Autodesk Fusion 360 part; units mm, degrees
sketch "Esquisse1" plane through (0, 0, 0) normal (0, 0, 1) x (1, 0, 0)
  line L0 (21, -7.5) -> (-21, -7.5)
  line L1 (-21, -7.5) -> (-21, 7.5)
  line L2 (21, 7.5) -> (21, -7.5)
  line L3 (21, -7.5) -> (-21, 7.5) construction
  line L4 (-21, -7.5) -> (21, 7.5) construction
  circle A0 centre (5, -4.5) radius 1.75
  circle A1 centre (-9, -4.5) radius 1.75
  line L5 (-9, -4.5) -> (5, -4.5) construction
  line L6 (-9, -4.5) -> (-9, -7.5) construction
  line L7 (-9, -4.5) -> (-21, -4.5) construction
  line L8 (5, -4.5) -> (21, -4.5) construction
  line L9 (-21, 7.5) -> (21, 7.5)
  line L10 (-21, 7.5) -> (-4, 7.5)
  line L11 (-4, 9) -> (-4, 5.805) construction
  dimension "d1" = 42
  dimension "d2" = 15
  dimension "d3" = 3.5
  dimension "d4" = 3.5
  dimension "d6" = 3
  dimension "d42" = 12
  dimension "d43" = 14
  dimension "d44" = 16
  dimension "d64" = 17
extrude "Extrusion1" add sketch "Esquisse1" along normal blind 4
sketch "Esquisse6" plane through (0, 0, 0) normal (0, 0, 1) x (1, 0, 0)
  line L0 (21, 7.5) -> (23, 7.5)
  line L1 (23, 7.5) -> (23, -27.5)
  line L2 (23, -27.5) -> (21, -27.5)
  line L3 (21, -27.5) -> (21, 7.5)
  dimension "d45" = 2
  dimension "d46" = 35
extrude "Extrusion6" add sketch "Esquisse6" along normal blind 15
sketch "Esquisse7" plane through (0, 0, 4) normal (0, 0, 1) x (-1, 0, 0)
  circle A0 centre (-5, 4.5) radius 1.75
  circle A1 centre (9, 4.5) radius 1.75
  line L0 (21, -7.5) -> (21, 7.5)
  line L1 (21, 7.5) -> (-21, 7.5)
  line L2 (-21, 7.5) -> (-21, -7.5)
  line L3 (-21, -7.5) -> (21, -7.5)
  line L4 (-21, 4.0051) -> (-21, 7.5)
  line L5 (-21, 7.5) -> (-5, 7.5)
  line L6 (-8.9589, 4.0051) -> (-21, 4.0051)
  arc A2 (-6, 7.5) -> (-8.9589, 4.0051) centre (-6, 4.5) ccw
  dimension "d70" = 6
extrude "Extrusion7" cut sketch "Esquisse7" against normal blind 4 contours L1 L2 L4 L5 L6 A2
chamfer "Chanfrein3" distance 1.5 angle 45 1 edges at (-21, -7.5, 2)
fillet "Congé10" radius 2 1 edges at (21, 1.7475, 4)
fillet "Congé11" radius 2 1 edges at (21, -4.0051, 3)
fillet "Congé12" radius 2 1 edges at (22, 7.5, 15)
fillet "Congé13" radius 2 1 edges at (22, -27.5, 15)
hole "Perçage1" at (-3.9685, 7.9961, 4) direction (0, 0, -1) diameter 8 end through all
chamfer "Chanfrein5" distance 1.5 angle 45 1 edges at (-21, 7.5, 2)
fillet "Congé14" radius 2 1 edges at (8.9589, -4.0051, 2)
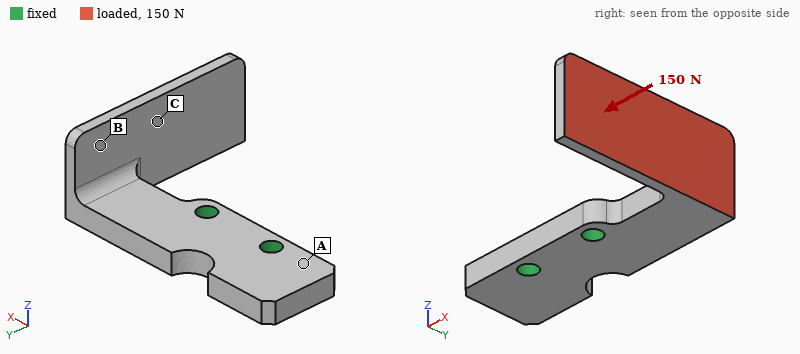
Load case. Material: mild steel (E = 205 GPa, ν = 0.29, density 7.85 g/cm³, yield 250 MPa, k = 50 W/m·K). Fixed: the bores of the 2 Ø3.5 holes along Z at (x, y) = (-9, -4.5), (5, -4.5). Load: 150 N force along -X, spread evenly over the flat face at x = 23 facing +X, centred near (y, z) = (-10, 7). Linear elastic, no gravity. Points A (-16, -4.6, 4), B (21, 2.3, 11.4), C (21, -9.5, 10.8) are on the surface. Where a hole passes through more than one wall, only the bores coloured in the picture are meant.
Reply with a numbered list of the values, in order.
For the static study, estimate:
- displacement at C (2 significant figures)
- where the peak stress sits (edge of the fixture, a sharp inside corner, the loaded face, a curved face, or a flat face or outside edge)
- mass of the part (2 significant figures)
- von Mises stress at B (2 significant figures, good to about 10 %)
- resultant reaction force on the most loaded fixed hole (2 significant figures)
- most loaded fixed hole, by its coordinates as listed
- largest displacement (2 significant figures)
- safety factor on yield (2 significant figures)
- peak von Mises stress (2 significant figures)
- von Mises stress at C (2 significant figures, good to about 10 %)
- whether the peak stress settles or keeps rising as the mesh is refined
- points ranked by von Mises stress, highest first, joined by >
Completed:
1. 0.037 mm
2. a curved face
3. 25 g
4. 32 MPa
5. 200 N
6. (5, -4.5)
7. 0.14 mm
8. 0.89
9. 280 MPa
10. 58 MPa
11. settles
12. C > B > A
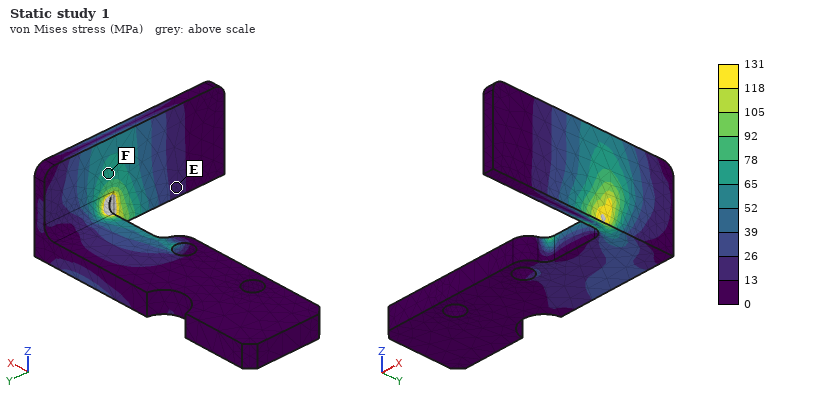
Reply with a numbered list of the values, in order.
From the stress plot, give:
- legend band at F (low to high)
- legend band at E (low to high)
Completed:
1. 65 to 78 MPa
2. 13 to 26 MPa
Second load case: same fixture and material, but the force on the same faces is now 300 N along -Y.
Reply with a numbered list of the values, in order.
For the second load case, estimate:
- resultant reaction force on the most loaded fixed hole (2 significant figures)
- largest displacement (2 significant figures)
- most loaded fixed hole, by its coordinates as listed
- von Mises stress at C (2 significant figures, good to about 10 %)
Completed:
1. 650 N
2. 71 µm
3. (5, -4.5)
4. 9.2 MPa
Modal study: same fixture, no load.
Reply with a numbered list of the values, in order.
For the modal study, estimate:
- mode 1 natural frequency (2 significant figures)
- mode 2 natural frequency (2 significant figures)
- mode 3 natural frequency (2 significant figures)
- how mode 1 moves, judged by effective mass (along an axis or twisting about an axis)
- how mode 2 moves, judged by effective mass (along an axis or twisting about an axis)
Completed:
1. 2300 Hz
2. 2900 Hz
3. 4800 Hz
4. along X
5. along Z
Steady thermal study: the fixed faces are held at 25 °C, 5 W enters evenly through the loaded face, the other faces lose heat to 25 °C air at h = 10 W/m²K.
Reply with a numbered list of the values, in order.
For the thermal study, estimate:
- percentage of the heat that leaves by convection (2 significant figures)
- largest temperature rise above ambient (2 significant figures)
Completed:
1. 9.8 %
2. 70 K
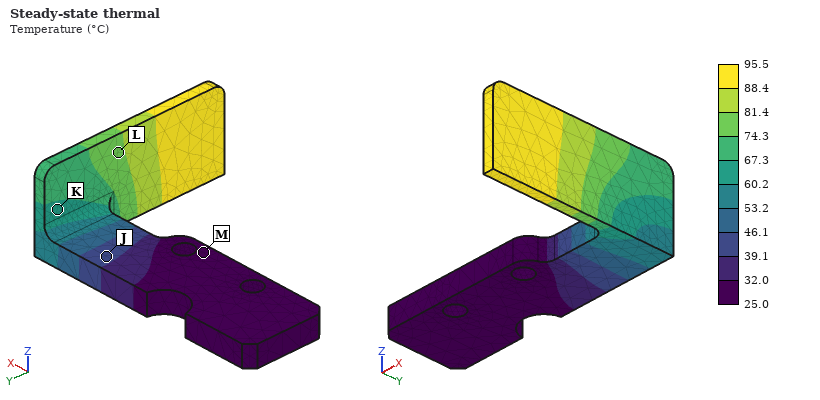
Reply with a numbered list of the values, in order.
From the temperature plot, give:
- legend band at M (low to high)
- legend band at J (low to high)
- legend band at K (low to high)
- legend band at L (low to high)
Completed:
1. 25.0 to 32.0 °C
2. 39.1 to 46.1 °C
3. 60.2 to 67.3 °C
4. 74.3 to 81.4 °C
